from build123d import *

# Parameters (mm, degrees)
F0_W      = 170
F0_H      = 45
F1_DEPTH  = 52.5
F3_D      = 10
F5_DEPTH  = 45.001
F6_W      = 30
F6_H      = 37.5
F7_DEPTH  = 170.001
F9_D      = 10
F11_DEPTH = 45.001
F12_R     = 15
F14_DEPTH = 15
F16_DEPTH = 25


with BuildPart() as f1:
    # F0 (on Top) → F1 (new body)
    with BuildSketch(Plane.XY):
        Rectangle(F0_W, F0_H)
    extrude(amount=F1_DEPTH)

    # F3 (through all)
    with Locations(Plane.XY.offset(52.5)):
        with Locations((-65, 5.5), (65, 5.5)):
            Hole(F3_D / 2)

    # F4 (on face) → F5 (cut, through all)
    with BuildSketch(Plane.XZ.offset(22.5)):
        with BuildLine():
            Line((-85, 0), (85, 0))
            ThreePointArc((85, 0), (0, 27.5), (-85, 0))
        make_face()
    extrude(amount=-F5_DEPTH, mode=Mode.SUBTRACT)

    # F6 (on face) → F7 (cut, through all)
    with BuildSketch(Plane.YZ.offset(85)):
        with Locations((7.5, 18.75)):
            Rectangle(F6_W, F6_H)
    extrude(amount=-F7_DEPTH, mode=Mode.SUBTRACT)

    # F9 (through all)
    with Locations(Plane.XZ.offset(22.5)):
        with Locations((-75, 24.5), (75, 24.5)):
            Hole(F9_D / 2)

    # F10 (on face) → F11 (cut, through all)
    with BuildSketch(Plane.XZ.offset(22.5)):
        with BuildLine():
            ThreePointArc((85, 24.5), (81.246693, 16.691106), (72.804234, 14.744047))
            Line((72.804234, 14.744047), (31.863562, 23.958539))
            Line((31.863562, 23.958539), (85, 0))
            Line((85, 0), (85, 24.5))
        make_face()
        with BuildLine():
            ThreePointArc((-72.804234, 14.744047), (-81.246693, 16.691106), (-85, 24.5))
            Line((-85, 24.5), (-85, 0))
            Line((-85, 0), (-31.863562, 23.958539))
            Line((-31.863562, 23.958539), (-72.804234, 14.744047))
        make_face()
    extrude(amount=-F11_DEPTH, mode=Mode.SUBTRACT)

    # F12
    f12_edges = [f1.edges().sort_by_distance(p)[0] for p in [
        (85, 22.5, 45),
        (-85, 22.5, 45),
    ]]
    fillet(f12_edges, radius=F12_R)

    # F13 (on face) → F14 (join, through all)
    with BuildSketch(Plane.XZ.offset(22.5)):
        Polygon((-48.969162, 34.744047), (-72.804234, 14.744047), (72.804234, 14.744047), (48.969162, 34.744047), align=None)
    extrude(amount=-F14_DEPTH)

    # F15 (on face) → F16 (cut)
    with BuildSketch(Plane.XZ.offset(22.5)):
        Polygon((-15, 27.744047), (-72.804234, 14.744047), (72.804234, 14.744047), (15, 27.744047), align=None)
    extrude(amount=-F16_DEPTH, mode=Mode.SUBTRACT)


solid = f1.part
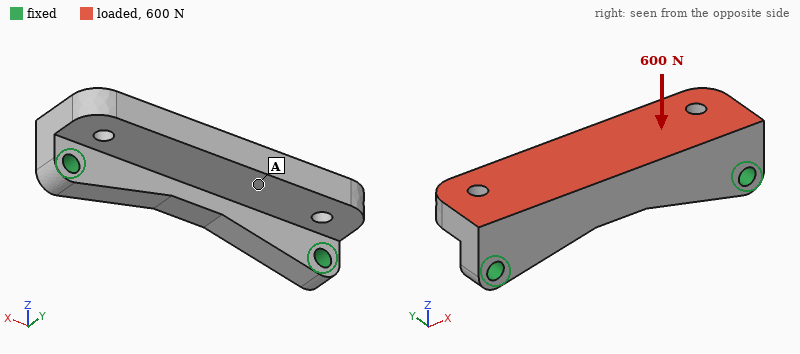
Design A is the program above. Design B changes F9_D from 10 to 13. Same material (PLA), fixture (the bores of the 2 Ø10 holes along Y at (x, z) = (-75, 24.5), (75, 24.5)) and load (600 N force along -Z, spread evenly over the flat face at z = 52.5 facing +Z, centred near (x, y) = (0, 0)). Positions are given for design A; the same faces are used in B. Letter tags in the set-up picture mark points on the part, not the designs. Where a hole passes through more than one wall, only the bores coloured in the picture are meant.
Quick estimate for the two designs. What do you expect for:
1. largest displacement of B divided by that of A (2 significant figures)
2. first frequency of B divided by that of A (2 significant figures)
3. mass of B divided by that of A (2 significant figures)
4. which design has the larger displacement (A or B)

0.89
1.1
0.99
A
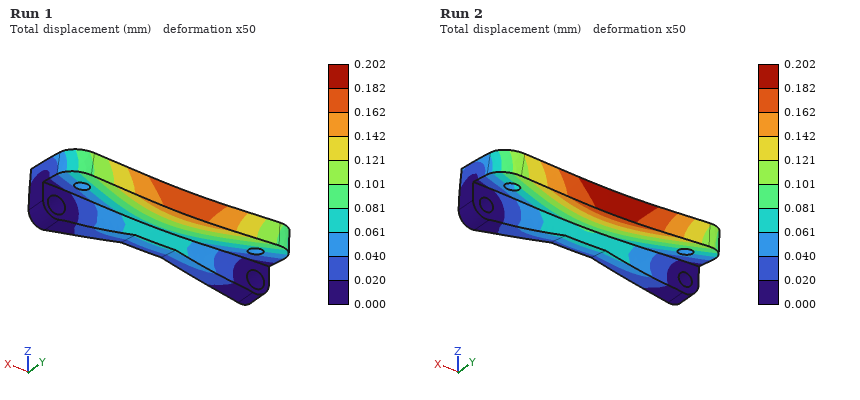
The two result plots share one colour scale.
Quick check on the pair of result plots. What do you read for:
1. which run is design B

Run 1
